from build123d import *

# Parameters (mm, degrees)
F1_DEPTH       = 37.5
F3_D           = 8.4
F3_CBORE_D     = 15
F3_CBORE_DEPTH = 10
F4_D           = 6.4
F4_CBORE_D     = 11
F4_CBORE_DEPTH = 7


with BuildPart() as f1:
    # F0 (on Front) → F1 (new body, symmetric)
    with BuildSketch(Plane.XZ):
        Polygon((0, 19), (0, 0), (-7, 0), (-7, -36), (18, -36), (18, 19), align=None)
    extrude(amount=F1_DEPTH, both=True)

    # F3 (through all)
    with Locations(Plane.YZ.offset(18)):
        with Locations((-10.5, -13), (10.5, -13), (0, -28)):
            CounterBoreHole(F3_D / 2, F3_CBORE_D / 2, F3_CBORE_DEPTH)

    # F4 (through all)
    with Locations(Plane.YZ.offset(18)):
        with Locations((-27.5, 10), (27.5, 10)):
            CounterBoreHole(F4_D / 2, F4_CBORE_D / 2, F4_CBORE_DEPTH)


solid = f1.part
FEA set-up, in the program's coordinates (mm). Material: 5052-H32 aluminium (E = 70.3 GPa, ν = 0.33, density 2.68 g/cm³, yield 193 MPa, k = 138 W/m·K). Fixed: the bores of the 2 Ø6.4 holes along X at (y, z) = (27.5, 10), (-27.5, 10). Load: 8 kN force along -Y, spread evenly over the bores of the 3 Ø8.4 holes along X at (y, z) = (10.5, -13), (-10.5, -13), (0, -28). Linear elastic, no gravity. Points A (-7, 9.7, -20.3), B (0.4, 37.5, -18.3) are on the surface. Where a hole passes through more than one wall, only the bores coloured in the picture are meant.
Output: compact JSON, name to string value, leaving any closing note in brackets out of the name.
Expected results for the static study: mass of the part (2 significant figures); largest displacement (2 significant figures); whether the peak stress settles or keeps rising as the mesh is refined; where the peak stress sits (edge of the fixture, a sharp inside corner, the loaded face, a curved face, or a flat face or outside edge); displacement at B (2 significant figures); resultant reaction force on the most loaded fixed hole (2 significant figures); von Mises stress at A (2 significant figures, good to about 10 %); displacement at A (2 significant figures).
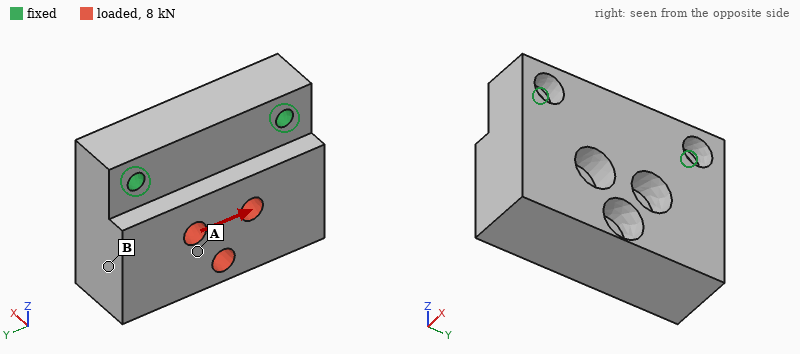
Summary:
{"mass of the part": "220 g", "largest displacement": "20 µm", "whether the peak stress settles or keeps rising as the mesh is refined": "keeps rising", "where the peak stress sits": "edge of the fixture", "displacement at B": "14 µm", "resultant reaction force on the most loaded fixed hole": "5.6 kN", "von Mises stress at A": "15 MPa", "displacement at A": "15 µm"}
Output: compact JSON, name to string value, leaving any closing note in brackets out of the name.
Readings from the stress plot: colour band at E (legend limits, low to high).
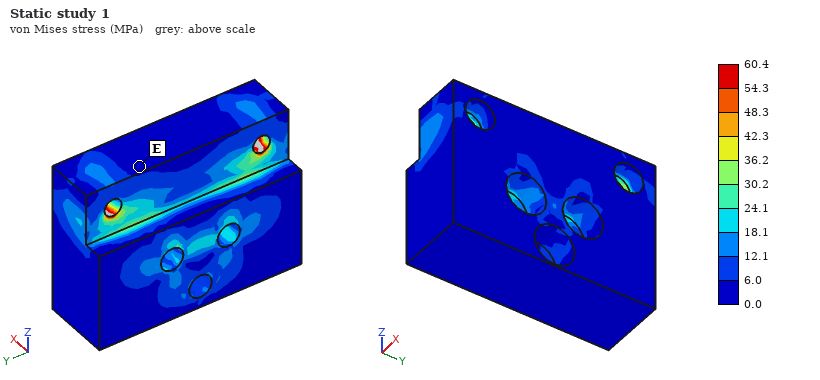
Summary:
{"colour band at E": "0.0 to 6.0 MPa"}
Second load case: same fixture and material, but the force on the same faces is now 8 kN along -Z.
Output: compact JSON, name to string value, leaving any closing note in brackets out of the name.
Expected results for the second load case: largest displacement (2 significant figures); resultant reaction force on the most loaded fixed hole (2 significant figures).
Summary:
{"largest displacement": "46 µm", "resultant reaction force on the most loaded fixed hole": "4.2 kN"}
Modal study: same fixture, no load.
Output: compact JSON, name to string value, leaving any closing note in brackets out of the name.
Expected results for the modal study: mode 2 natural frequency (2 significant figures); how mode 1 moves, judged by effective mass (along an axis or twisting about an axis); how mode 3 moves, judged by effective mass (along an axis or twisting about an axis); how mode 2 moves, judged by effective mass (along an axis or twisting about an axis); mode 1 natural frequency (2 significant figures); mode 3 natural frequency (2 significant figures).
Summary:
{"mode 2 natural frequency": "7700 Hz", "how mode 1 moves, judged by effective mass": "along X", "how mode 3 moves, judged by effective mass": "along Y", "how mode 2 moves, judged by effective mass": "twisting about Z", "mode 1 natural frequency": "3200 Hz", "mode 3 natural frequency": "9800 Hz"}
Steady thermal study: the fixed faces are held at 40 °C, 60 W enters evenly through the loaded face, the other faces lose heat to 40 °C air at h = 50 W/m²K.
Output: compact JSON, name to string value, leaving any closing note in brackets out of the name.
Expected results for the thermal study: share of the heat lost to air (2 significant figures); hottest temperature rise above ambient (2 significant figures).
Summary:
{"share of the heat lost to air": "10 %", "hottest temperature rise above ambient": "15 K"}
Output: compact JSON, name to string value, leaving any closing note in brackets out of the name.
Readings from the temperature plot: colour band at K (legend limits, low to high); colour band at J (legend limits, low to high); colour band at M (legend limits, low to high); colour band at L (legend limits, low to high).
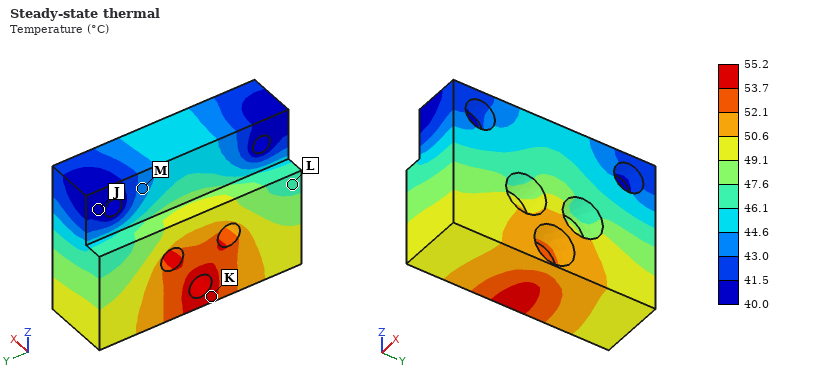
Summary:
{"colour band at K": "53.7 to 55.2 °C", "colour band at J": "40.0 to 41.5 °C", "colour band at M": "43.0 to 44.6 °C", "colour band at L": "46.1 to 47.6 °C"}
